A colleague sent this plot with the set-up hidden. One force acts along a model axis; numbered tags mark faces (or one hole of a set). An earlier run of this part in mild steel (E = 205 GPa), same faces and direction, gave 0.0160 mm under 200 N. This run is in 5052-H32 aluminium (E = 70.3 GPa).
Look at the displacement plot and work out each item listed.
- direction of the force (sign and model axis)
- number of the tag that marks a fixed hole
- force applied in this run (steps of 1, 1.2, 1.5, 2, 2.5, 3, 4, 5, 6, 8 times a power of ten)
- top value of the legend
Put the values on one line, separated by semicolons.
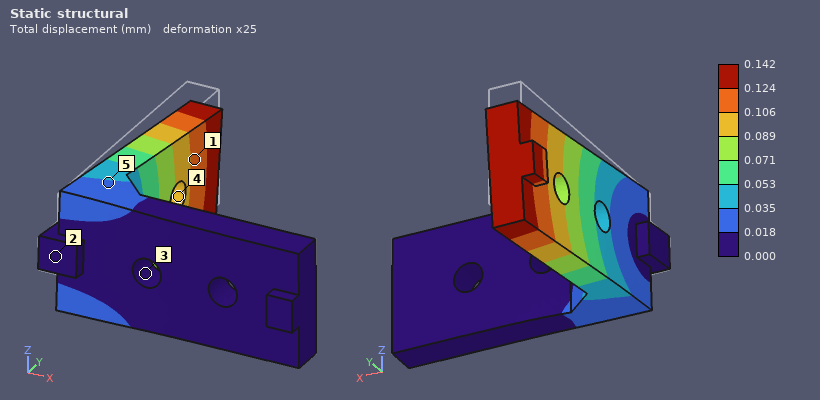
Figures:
-Z; 3; 600 N; 0.142 mm
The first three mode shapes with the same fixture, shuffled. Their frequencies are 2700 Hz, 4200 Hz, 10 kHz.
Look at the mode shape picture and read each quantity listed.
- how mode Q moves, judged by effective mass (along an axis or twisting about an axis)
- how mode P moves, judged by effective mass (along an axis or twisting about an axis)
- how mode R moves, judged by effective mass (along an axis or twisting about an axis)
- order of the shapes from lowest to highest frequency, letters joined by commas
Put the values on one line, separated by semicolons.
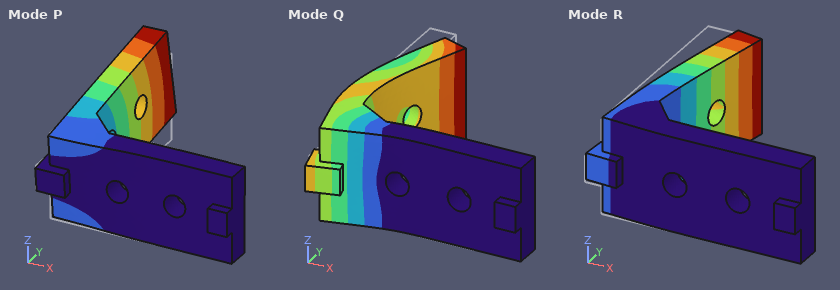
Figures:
along Y; along Z; along X; R, P, Q
